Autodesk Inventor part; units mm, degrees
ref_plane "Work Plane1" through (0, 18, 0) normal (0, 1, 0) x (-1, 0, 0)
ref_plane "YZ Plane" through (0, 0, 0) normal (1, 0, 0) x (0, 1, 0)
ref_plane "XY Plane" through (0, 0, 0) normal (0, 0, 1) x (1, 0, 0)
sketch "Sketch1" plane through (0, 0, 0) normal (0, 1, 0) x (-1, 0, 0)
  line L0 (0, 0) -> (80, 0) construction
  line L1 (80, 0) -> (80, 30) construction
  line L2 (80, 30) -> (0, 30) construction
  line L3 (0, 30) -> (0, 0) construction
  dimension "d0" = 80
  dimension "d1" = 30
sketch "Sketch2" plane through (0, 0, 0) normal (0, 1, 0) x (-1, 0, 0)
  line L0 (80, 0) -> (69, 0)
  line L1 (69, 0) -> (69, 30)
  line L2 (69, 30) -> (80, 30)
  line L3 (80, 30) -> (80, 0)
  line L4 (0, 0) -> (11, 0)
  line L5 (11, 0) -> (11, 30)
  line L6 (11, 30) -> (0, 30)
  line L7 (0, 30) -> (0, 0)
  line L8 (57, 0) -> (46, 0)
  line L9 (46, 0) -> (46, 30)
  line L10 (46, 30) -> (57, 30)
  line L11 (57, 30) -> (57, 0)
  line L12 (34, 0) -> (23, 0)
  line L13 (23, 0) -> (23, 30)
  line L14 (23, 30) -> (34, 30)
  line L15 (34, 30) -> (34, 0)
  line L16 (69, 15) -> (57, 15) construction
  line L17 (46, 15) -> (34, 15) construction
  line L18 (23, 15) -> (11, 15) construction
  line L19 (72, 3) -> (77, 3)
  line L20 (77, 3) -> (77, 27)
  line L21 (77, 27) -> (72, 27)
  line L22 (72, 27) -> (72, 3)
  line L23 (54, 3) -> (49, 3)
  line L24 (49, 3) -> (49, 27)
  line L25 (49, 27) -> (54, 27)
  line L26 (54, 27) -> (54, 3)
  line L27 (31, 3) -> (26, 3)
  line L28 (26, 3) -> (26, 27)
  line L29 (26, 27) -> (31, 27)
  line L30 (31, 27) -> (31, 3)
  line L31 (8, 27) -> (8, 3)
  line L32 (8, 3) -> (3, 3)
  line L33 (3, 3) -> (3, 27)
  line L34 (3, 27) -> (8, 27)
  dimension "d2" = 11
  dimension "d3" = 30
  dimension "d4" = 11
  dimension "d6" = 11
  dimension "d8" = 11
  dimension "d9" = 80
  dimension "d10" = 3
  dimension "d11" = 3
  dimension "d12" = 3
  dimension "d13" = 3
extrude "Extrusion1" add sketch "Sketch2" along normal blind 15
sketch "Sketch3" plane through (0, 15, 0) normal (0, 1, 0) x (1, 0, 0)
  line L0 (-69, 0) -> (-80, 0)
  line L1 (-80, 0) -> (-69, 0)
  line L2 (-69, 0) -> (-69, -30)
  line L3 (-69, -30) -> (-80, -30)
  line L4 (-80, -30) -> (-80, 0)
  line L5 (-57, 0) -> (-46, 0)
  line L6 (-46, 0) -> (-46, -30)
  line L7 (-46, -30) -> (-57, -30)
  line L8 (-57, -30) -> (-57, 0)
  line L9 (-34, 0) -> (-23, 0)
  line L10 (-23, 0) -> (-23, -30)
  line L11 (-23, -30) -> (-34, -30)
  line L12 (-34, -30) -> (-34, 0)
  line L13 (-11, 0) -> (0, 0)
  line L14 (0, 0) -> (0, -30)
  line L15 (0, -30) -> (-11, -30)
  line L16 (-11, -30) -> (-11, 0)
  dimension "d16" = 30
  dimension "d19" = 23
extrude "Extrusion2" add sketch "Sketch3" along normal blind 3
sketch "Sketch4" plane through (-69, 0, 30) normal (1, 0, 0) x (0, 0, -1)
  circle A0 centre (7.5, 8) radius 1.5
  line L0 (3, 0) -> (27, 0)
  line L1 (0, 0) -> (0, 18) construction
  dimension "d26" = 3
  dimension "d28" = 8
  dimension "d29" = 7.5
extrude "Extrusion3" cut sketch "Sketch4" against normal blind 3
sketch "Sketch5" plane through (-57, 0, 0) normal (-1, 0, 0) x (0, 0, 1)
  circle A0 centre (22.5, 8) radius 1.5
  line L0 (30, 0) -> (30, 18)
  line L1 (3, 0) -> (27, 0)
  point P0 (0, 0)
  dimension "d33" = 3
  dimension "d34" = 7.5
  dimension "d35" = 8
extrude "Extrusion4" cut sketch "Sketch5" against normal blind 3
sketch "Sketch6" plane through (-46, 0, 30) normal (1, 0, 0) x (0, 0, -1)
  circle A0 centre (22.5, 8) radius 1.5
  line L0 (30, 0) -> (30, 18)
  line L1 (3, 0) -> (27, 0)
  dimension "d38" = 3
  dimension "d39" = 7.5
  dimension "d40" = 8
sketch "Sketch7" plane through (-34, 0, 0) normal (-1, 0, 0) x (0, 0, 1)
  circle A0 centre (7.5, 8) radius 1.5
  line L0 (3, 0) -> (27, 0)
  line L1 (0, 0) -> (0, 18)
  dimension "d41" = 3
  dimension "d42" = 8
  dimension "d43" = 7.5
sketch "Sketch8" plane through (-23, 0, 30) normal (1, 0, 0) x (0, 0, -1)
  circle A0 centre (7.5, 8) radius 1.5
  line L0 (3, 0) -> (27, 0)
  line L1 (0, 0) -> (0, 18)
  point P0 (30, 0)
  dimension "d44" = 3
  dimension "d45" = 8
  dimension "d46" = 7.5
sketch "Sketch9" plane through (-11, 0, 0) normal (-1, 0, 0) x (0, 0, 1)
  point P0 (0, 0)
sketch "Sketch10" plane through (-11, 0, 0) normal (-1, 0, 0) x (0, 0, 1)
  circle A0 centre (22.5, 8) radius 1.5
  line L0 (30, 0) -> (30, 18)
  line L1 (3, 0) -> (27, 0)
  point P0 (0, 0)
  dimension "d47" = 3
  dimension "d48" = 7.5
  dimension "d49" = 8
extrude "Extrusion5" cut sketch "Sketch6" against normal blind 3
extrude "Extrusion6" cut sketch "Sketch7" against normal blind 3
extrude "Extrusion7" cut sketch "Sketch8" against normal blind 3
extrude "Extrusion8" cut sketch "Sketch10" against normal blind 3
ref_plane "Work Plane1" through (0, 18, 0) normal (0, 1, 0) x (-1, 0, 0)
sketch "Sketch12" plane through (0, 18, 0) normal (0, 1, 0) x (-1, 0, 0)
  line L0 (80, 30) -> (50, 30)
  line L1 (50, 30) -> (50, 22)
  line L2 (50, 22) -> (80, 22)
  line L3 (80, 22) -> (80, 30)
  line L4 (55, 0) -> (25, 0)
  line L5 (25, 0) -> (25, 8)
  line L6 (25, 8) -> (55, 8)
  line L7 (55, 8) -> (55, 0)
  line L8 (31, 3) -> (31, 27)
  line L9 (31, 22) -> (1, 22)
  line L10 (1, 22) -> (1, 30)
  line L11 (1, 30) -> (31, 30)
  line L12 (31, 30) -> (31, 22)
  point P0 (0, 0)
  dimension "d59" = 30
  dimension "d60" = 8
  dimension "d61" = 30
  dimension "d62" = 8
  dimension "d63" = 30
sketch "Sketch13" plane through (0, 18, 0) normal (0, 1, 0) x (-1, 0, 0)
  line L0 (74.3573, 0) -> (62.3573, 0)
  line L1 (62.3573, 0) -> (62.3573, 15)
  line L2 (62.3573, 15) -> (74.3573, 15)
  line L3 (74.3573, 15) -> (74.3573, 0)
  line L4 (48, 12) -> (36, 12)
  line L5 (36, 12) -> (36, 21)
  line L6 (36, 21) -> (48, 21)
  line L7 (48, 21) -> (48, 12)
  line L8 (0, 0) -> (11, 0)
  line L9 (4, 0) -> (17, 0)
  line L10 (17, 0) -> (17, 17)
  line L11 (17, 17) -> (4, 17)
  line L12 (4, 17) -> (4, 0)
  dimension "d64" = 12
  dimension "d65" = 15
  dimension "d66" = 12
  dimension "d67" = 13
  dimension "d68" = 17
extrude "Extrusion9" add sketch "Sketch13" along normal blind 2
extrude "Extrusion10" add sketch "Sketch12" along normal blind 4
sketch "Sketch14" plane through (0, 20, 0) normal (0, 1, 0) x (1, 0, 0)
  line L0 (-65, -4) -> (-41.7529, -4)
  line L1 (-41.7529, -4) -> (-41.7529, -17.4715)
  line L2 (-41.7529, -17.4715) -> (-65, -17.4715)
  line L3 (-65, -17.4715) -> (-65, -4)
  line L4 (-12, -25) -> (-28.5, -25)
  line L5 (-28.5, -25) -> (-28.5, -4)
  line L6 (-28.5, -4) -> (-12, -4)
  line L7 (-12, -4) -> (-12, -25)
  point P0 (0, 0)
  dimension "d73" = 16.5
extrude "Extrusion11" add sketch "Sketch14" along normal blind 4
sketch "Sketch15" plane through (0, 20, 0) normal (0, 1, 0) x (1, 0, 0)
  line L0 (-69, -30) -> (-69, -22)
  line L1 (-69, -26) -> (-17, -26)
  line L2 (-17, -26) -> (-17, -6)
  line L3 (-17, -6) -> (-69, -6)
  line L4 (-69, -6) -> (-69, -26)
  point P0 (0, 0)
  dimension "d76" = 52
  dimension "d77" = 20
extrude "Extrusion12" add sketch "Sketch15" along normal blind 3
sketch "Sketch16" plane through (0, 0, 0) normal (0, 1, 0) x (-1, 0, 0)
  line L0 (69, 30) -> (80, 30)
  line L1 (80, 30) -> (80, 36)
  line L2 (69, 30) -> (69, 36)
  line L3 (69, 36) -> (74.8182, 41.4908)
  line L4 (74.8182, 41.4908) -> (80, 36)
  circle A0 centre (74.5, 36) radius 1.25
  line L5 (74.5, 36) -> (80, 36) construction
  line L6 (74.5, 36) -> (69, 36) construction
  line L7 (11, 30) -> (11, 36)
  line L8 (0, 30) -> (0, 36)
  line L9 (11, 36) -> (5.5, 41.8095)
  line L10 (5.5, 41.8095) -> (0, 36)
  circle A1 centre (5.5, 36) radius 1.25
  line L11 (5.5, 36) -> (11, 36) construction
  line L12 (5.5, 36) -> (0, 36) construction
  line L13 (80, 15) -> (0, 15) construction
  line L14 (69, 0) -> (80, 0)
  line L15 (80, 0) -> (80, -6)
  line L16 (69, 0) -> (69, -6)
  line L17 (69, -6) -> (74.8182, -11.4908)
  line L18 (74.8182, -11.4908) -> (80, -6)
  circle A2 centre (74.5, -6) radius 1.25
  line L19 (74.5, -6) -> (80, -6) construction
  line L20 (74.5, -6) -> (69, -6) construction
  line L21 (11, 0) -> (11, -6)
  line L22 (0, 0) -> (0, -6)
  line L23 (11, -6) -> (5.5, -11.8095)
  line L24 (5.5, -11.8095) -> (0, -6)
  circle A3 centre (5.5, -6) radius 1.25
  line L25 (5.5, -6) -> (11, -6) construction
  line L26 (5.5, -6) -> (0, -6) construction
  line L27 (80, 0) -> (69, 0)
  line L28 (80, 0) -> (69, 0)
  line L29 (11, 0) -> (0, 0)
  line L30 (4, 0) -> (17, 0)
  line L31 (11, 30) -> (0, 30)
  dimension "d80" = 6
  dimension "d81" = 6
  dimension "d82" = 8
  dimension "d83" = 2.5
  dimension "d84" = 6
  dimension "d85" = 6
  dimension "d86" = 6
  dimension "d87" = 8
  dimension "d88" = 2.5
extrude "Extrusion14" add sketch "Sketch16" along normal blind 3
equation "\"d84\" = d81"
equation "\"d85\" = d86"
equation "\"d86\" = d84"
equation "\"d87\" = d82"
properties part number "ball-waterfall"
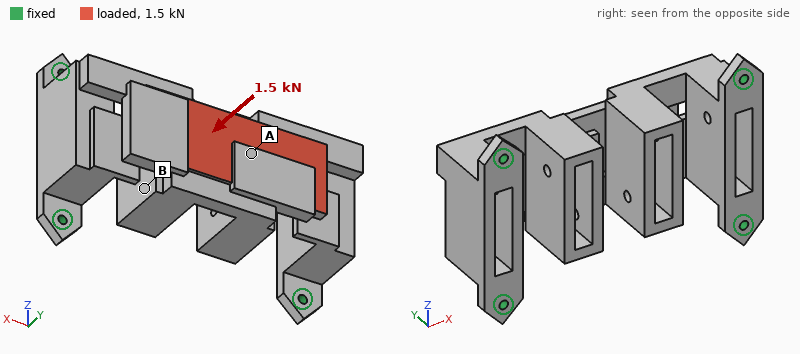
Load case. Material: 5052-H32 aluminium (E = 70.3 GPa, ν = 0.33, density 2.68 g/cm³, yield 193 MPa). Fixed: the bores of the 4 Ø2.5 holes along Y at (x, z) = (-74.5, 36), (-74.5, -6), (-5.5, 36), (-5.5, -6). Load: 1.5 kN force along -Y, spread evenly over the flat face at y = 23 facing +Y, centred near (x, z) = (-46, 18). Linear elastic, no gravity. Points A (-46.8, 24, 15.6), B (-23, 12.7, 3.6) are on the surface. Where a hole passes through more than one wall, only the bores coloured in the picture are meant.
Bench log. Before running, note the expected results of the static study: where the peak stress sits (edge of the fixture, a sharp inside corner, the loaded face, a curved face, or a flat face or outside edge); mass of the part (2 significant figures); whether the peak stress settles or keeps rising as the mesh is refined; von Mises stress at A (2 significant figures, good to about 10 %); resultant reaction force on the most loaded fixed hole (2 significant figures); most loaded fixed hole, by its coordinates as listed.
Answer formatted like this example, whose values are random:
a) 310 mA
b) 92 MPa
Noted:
a) edge of the fixture
b) 68 g
c) keeps rising
d) 55 MPa
e) 650 N
f) (-74.5, 36)
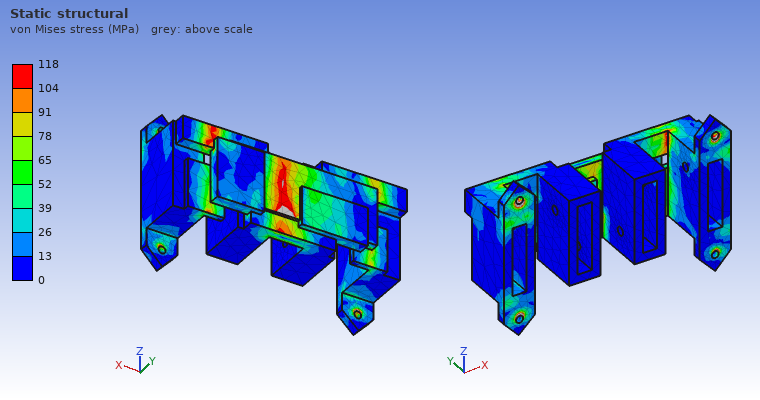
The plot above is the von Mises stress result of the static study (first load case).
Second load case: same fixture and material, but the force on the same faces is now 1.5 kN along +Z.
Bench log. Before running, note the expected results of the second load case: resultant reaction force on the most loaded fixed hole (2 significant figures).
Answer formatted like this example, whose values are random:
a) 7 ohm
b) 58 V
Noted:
a) 700 N
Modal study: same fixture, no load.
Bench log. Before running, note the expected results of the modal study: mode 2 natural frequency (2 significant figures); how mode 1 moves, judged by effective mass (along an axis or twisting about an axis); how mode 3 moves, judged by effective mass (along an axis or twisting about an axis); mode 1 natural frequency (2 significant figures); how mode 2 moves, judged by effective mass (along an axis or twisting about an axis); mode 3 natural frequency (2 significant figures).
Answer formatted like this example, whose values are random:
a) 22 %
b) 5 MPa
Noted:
a) 2500 Hz
b) along X
c) along Z
d) 1900 Hz
e) along Y
f) 3500 Hz
